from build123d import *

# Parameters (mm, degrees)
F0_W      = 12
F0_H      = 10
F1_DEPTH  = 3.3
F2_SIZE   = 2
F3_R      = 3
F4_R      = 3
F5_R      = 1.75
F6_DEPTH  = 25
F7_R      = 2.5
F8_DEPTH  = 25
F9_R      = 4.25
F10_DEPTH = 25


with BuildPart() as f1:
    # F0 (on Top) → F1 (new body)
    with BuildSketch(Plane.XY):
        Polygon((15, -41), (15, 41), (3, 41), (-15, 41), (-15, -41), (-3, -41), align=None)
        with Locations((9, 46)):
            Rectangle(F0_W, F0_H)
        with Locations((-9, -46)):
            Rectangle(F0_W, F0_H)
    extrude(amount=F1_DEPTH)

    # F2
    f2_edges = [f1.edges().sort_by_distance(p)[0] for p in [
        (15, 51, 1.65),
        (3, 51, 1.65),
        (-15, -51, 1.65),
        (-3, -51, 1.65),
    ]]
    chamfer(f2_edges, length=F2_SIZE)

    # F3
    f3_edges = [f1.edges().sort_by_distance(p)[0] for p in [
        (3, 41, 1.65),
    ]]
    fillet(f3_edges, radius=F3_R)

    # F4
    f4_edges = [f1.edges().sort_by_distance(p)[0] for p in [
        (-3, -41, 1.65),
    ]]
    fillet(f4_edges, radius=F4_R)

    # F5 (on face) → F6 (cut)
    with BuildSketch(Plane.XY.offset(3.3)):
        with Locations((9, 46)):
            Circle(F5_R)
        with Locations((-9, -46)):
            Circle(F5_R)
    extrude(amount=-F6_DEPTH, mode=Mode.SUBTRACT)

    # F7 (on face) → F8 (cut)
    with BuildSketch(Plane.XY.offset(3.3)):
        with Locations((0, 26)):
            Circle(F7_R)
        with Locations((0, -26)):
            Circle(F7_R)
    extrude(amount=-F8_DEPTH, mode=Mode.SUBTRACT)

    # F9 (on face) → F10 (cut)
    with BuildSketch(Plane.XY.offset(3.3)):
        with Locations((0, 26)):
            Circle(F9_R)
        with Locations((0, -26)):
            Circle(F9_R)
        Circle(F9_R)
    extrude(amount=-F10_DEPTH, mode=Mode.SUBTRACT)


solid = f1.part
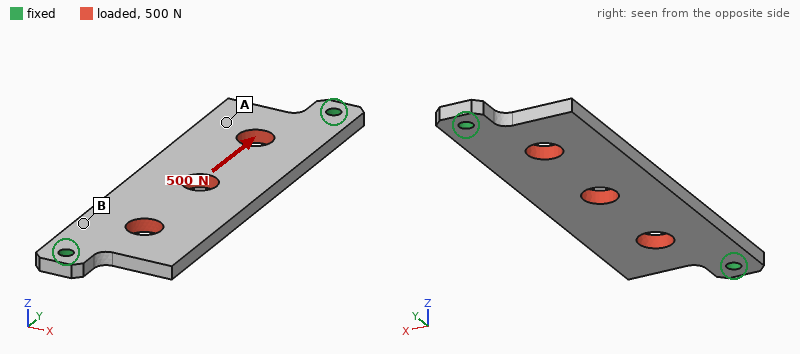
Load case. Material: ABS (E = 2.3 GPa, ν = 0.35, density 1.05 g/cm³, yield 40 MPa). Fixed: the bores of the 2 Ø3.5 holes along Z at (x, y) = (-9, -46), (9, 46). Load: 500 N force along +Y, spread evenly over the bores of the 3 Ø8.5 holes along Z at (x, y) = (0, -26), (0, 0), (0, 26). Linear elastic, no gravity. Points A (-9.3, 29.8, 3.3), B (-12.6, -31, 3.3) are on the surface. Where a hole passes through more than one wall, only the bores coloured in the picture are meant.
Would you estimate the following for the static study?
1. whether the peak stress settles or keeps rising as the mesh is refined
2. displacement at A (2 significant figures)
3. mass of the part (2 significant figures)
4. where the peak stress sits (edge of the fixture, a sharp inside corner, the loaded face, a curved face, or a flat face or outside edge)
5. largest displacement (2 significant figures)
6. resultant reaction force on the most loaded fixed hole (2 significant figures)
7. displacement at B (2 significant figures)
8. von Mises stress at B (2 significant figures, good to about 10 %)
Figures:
keeps rising
0.13 mm
8.7 g
edge of the fixture
0.15 mm
250 N
0.058 mm
5.4 MPa
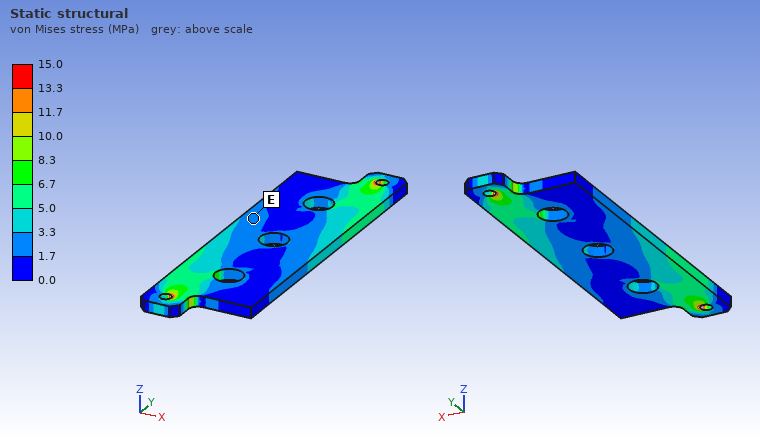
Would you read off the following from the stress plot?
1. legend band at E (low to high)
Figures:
1.7 to 3.3 MPa
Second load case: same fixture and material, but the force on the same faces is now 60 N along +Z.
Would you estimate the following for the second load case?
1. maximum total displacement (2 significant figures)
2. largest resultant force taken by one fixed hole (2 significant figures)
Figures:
1.2 mm
30 N
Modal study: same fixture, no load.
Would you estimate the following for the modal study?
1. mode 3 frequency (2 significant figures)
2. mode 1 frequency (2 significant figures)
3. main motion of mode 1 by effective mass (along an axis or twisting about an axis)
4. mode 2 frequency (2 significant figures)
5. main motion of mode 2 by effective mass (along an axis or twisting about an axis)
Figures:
1400 Hz
460 Hz
along Z
690 Hz
twisting about Y
